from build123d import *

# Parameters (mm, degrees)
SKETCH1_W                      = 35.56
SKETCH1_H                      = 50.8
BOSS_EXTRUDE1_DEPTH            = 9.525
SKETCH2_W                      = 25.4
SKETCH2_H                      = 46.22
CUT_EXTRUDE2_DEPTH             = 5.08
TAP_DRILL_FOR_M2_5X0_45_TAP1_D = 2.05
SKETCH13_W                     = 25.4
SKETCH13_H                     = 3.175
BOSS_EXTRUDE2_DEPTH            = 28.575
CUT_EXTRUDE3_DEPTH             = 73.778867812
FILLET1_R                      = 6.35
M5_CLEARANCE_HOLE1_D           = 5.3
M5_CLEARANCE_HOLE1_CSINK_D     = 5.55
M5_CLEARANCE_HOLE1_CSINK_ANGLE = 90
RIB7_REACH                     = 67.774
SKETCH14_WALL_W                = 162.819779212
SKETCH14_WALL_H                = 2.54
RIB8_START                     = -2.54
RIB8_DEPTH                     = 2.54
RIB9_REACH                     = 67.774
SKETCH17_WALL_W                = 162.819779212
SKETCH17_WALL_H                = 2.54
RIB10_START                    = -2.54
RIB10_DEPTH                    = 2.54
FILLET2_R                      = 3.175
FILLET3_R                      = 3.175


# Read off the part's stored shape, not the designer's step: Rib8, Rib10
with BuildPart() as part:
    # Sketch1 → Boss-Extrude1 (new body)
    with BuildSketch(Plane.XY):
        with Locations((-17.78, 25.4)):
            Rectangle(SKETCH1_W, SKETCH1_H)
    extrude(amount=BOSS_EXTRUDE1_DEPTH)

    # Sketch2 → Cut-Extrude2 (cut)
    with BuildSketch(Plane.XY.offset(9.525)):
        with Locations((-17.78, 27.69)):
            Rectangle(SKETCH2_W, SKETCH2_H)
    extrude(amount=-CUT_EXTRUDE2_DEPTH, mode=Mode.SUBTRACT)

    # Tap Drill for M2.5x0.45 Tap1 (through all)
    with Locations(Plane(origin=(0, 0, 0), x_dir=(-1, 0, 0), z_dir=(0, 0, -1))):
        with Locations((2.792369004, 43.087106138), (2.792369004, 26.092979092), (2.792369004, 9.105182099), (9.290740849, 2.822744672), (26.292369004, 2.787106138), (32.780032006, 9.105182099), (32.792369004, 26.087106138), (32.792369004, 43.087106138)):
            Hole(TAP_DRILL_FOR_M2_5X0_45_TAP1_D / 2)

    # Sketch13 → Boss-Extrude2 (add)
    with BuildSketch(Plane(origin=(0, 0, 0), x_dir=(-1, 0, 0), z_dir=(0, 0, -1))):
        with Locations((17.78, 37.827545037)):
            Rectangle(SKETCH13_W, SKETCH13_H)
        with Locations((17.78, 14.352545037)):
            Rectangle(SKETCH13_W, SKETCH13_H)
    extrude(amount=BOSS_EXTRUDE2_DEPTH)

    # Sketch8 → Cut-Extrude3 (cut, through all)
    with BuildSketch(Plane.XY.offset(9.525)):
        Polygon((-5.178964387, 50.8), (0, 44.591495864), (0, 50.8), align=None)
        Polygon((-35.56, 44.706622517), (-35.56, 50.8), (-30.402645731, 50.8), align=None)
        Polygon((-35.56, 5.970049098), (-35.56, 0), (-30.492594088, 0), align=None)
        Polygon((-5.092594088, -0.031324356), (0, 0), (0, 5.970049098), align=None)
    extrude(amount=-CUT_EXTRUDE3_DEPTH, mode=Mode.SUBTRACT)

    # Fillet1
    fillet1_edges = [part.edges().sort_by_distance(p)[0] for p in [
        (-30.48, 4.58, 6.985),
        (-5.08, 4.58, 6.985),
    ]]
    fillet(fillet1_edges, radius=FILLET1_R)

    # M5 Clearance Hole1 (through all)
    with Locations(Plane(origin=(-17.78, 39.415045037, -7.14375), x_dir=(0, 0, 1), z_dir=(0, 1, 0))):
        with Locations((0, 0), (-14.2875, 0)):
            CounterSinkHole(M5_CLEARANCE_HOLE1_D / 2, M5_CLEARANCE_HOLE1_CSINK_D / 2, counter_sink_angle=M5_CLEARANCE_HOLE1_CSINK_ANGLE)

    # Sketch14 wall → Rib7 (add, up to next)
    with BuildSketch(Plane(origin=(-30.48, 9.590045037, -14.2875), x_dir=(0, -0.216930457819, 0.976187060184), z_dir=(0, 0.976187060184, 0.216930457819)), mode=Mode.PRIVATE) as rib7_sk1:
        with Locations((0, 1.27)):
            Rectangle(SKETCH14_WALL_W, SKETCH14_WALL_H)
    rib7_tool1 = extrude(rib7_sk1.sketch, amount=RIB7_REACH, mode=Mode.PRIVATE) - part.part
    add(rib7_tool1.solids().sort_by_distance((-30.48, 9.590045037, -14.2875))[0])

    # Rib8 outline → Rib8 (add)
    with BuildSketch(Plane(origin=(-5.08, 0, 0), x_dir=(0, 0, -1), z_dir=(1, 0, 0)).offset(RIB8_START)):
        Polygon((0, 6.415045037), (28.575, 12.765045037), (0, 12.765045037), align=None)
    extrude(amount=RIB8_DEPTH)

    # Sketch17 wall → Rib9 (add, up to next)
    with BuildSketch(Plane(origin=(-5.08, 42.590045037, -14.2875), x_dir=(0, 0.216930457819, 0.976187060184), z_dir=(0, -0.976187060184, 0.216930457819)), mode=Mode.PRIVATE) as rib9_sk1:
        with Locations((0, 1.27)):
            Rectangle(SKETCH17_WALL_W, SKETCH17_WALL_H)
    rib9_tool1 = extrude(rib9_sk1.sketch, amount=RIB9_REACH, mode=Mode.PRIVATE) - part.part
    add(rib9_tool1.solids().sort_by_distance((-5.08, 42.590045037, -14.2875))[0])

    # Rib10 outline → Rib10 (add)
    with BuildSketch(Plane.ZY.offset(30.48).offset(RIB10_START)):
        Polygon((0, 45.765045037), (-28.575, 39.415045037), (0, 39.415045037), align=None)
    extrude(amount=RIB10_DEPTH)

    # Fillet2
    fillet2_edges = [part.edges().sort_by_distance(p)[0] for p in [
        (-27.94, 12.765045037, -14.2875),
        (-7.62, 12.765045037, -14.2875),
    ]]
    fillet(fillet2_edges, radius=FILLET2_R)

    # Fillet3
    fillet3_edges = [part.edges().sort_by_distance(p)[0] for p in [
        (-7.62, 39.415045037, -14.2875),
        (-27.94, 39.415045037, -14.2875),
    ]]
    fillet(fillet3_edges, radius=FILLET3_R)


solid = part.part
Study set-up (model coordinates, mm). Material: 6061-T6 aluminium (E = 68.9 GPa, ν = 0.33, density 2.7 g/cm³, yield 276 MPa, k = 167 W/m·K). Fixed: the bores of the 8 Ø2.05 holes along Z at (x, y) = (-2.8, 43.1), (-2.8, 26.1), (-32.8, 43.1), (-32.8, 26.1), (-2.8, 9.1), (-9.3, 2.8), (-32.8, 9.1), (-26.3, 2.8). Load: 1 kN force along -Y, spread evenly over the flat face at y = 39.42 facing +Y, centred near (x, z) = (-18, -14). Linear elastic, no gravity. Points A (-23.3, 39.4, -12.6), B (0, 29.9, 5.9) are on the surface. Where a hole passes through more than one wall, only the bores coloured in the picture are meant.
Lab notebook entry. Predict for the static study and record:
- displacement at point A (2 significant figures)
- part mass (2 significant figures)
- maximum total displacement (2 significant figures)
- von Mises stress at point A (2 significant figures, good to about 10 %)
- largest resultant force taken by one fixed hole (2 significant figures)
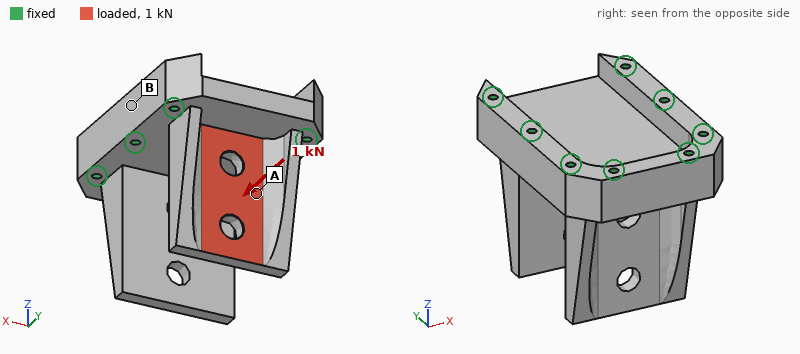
0.061 mm
43 g
0.19 mm
33 MPa
500 N
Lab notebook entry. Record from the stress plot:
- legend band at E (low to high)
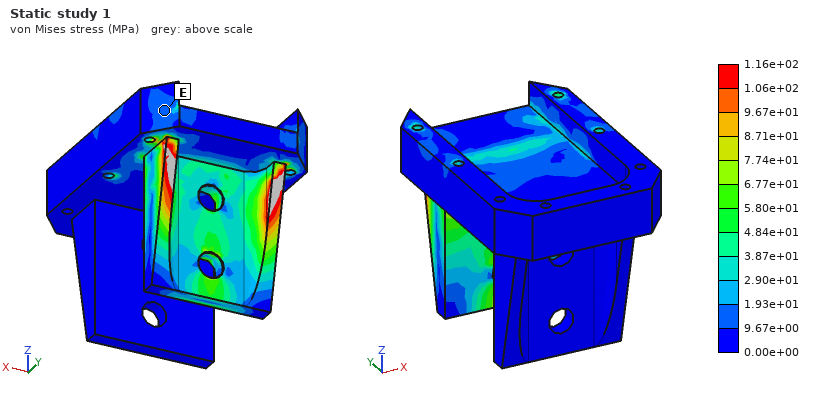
9.67e+00 to 1.93e+01 MPa
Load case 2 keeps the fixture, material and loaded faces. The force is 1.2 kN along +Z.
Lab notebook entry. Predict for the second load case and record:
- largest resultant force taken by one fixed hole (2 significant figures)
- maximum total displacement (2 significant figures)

490 N
14 µm
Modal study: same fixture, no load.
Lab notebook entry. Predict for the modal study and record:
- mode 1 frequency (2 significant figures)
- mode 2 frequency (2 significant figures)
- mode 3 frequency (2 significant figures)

5900 Hz
6100 Hz
10 kHz
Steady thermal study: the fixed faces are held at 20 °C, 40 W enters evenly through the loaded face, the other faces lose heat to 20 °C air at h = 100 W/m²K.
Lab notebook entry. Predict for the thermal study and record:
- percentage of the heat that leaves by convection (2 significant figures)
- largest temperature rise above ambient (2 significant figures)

14 %
43 K
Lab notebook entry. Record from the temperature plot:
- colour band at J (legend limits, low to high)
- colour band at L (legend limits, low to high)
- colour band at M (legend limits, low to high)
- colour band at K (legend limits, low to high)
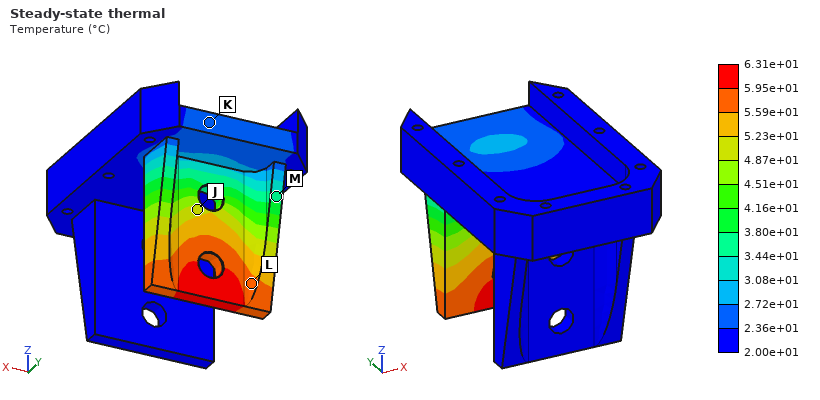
4.87e+01 to 5.23e+01 °C
5.59e+01 to 5.95e+01 °C
3.44e+01 to 3.80e+01 °C
2.36e+01 to 2.72e+01 °C
